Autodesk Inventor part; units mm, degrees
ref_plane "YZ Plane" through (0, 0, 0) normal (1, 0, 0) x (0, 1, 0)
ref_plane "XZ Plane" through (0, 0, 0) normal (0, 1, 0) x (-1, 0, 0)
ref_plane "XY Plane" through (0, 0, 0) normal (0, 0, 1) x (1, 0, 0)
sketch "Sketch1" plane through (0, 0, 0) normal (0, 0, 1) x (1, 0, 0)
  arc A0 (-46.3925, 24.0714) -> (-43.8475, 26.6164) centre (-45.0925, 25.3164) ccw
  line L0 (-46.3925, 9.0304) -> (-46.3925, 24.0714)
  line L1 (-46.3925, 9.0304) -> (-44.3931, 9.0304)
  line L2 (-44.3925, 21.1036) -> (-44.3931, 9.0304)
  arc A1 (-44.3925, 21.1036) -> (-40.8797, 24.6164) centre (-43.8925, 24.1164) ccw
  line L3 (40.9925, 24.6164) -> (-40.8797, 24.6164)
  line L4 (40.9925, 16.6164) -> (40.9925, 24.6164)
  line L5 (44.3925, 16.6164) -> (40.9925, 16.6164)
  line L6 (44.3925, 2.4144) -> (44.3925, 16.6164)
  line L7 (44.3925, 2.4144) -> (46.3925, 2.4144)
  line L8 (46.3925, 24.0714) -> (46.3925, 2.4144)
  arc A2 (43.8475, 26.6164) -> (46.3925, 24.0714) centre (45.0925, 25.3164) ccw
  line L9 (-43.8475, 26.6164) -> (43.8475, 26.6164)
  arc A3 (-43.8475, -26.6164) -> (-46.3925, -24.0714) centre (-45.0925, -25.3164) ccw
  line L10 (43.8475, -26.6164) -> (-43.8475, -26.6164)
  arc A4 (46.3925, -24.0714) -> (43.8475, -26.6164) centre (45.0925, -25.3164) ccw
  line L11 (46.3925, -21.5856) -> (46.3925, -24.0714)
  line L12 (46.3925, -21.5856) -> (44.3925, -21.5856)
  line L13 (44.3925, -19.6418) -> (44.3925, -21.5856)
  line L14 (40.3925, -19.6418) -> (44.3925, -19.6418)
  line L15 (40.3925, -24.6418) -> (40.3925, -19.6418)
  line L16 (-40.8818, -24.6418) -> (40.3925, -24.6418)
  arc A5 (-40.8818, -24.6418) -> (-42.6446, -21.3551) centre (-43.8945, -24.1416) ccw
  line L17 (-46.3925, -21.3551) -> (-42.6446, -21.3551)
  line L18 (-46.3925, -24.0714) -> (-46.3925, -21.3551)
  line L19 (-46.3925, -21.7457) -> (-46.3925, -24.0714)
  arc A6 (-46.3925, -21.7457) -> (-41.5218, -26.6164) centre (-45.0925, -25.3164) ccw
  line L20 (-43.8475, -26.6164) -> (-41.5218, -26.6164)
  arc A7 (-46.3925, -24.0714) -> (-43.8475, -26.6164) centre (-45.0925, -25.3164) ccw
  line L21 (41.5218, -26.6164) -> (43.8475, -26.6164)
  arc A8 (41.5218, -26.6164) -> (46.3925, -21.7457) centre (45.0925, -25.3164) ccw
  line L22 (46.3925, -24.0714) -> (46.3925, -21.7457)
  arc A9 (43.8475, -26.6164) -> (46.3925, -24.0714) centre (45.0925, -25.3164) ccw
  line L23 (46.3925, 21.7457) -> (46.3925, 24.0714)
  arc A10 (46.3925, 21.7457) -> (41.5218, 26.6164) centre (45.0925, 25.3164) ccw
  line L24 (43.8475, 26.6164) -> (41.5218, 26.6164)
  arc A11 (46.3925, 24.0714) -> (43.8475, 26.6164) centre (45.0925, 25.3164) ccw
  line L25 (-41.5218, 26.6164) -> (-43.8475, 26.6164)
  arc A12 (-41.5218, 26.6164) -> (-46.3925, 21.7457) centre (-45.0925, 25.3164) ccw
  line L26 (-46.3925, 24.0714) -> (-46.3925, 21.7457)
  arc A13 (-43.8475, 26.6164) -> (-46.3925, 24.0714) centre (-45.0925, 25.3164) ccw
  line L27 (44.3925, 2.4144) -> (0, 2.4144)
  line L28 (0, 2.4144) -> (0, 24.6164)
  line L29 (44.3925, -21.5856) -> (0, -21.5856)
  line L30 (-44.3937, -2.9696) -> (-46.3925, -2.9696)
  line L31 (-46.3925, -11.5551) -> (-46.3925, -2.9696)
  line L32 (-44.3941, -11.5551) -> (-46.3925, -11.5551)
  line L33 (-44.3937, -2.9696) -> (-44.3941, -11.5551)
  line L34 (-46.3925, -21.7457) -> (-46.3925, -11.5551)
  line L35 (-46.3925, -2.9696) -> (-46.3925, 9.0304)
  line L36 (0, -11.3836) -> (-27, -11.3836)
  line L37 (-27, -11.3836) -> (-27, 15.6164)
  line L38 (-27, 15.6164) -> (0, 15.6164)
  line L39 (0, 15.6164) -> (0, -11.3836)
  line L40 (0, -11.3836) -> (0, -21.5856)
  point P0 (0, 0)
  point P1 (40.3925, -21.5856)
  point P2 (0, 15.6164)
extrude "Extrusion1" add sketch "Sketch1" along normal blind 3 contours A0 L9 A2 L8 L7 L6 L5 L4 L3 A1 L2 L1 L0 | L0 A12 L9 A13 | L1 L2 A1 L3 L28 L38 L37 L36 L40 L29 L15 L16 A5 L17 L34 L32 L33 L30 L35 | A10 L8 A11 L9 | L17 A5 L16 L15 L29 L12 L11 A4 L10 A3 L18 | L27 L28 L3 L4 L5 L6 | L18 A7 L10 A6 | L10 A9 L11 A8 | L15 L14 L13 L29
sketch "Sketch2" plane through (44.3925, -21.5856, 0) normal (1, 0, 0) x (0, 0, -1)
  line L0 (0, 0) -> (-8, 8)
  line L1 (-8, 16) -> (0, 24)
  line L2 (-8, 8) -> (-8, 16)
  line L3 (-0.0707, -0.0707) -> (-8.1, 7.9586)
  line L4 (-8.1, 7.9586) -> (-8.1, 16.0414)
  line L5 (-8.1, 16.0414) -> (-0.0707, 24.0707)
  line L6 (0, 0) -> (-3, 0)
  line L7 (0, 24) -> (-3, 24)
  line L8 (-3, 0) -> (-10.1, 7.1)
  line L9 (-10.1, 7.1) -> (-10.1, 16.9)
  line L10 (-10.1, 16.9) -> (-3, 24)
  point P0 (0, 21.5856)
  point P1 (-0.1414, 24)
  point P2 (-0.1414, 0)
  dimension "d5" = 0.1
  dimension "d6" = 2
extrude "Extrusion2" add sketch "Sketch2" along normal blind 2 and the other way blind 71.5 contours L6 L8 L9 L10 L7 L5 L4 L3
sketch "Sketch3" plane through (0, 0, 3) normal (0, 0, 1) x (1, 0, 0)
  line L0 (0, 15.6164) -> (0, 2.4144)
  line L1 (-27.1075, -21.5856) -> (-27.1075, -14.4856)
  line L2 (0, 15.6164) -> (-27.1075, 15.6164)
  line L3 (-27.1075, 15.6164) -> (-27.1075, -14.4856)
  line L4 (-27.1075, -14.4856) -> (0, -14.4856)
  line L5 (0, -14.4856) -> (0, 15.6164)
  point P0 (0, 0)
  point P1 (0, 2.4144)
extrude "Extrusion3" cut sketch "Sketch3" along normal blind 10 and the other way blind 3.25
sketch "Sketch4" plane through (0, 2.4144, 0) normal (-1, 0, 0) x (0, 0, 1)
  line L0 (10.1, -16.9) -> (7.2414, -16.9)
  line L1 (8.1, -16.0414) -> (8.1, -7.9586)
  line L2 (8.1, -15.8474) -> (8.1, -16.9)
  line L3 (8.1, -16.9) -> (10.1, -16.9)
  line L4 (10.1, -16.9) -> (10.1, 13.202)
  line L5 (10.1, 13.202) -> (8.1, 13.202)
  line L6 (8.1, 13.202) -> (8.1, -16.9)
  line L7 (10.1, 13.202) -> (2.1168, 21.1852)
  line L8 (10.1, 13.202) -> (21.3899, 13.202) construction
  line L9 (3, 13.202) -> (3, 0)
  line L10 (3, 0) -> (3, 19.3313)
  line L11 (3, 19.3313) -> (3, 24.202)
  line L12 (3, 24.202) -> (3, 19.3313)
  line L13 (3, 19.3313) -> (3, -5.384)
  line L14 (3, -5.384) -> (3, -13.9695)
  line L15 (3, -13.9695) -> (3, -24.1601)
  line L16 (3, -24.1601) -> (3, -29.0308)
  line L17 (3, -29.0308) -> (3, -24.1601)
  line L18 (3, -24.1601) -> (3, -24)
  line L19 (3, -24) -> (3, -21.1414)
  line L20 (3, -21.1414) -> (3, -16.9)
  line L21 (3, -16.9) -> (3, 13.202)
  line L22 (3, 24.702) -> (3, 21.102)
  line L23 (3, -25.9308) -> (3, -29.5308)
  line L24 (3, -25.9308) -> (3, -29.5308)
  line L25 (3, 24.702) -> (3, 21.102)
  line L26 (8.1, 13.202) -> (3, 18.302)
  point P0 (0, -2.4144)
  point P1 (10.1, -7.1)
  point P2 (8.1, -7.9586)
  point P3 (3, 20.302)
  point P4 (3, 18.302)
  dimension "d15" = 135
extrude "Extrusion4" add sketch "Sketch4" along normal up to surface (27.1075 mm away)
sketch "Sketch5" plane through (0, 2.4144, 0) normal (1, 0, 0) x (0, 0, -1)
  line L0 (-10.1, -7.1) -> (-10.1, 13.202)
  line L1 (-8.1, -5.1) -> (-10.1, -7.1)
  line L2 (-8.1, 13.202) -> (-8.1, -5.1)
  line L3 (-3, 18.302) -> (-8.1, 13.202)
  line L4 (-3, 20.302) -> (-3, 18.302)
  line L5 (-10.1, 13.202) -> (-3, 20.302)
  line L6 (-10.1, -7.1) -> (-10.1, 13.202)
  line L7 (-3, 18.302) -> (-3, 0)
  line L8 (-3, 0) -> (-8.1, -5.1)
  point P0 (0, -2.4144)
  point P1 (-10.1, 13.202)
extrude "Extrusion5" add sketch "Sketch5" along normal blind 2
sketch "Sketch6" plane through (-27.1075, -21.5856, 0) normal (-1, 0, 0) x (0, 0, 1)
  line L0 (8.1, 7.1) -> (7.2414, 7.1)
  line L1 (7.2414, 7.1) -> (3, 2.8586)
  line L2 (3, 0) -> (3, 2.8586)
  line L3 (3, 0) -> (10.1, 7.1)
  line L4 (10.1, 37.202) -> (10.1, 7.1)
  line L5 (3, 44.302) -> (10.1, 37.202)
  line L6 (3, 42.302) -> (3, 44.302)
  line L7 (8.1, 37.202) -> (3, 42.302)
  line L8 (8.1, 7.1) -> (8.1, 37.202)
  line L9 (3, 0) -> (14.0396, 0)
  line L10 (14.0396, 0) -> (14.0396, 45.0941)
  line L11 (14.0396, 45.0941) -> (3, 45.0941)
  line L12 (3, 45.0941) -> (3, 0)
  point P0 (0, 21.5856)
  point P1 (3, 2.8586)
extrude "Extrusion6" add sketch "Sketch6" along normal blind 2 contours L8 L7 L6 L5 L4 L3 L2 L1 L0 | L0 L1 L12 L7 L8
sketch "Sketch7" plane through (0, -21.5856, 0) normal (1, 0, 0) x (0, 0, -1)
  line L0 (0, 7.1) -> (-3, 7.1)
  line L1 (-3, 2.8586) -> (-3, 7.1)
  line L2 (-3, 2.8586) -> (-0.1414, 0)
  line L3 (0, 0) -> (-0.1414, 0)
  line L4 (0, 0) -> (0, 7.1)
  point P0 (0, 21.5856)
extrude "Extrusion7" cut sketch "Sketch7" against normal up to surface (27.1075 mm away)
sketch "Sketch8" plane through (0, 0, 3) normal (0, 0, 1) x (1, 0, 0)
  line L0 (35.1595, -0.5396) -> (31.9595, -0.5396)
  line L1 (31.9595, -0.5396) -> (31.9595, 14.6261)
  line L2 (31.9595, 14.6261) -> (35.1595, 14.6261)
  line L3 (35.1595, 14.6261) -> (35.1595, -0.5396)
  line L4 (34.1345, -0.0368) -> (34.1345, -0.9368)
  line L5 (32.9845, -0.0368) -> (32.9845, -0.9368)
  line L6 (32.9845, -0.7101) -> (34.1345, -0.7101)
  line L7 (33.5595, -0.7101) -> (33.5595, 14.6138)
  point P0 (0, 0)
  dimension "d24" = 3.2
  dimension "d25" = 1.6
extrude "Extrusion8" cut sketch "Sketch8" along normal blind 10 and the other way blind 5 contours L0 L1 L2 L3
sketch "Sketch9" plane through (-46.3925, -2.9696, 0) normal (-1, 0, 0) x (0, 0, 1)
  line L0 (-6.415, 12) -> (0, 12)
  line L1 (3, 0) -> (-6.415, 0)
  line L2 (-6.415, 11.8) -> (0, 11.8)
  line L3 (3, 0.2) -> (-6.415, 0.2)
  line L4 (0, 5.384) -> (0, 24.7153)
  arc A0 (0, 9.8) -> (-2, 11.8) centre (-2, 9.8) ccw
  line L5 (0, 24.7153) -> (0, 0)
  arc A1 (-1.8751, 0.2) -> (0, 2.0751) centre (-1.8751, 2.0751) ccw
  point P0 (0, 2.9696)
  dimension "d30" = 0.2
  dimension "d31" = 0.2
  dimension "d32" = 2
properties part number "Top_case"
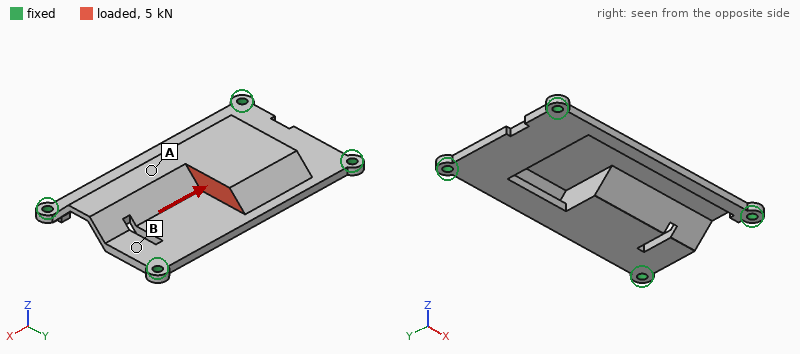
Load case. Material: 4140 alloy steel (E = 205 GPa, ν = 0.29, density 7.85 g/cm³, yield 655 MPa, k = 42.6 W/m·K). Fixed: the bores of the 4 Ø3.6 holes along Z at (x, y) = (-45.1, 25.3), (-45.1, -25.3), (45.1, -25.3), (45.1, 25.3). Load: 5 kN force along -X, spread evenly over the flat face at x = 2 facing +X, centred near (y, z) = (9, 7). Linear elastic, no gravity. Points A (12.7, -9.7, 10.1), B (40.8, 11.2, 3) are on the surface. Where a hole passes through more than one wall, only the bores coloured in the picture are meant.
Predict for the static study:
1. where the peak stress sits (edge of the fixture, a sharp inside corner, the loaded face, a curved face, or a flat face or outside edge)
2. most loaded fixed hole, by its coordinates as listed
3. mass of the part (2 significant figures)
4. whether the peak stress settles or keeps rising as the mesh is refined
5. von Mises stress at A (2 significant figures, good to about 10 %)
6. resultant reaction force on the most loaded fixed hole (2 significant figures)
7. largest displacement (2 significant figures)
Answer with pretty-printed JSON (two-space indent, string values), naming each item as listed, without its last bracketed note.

{
  "where the peak stress sits": "edge of the fixture",
  "most loaded fixed hole, by its coordinates as listed": "(-45.1, 25.3)",
  "mass of the part": "110 g",
  "whether the peak stress settles or keeps rising as the mesh is refined": "keeps rising",
  "von Mises stress at A": "39 MPa",
  "resultant reaction force on the most loaded fixed hole": "1.5 kN",
  "largest displacement": "75 µm"
}
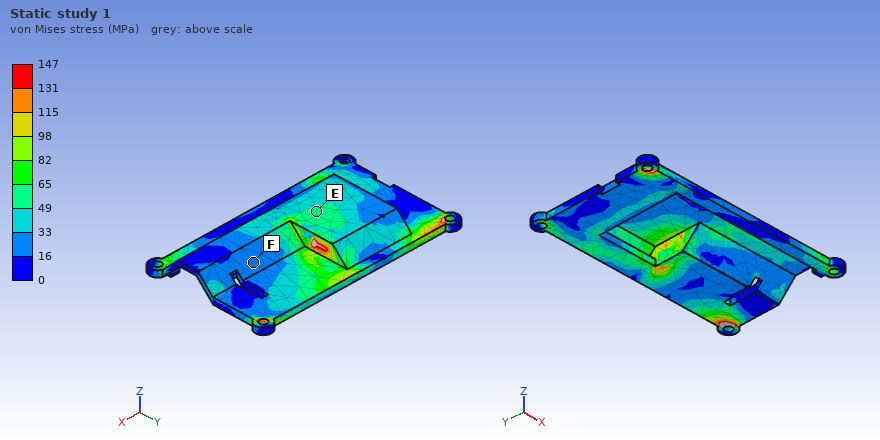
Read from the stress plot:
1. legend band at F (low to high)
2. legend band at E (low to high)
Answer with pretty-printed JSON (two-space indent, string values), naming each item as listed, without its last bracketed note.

{
  "legend band at F": "16 to 33 MPa",
  "legend band at E": "49 to 65 MPa"
}
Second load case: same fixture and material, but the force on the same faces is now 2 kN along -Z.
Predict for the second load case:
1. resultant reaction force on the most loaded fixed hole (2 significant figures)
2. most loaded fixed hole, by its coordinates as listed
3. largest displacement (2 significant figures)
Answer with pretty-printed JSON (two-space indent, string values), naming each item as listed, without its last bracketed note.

{
  "resultant reaction force on the most loaded fixed hole": "1.8 kN",
  "most loaded fixed hole, by its coordinates as listed": "(45.1, -25.3)",
  "largest displacement": "0.32 mm"
}
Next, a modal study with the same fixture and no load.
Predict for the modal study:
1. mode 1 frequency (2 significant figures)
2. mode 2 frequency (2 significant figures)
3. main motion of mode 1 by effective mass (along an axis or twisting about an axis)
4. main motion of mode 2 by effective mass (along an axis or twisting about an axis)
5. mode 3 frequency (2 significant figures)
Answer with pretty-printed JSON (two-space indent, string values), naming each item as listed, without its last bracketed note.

{
  "mode 1 frequency": "2400 Hz",
  "mode 2 frequency": "3600 Hz",
  "main motion of mode 1 by effective mass": "along Z",
  "main motion of mode 2 by effective mass": "along Z",
  "mode 3 frequency": "4700 Hz"
}
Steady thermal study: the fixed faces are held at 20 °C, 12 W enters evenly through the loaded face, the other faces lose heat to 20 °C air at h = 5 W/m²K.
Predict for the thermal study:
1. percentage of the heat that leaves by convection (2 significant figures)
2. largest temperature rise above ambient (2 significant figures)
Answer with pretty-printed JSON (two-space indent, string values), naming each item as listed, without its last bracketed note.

{
  "percentage of the heat that leaves by convection": "17 %",
  "largest temperature rise above ambient": "75 K"
}
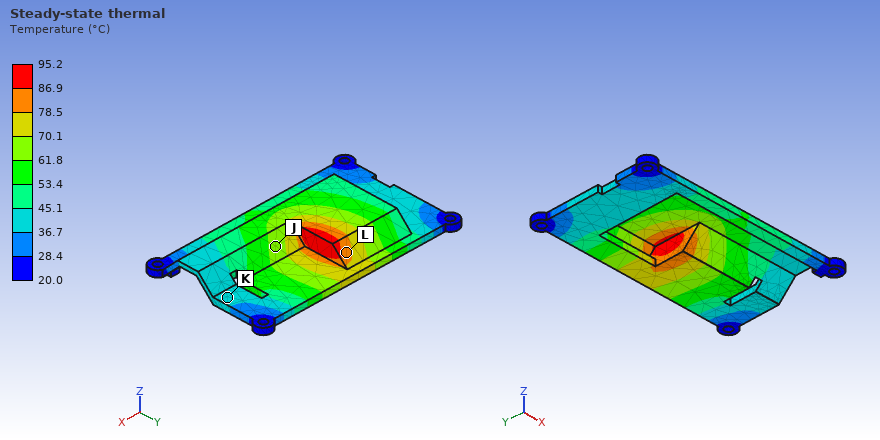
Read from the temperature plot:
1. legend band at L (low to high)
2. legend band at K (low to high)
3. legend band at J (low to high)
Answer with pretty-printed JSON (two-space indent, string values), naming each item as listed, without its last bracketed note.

{
  "legend band at L": "78.5 to 86.9 °C",
  "legend band at K": "36.7 to 45.1 °C",
  "legend band at J": "61.8 to 70.1 °C"
}
